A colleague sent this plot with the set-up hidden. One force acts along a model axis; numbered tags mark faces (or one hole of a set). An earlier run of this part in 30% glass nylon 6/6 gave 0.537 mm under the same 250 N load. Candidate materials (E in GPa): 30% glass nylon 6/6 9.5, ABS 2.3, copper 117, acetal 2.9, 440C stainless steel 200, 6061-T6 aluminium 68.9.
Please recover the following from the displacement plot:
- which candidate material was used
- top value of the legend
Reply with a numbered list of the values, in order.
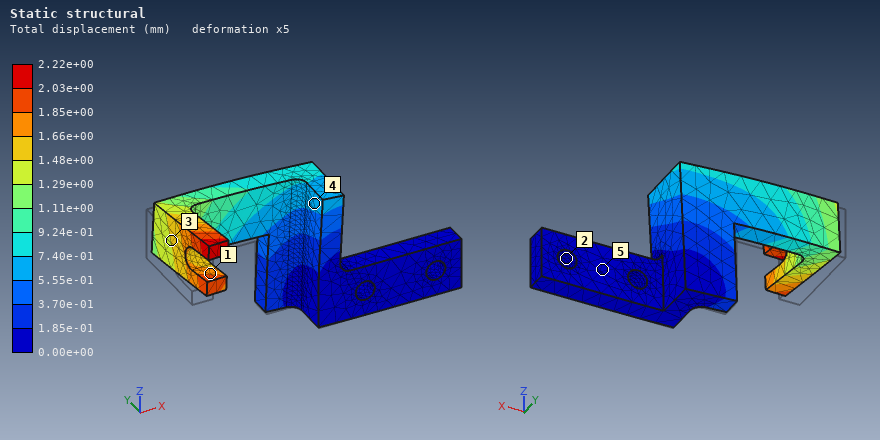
1. ABS
2. 2.22e+00 mm
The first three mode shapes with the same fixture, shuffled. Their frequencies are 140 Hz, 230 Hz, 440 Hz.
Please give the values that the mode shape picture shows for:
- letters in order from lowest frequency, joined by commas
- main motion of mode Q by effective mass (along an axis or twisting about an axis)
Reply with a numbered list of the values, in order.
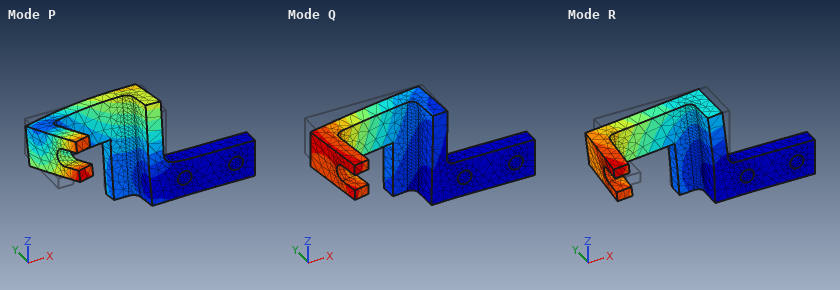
1. Q, R, P
2. along Y
